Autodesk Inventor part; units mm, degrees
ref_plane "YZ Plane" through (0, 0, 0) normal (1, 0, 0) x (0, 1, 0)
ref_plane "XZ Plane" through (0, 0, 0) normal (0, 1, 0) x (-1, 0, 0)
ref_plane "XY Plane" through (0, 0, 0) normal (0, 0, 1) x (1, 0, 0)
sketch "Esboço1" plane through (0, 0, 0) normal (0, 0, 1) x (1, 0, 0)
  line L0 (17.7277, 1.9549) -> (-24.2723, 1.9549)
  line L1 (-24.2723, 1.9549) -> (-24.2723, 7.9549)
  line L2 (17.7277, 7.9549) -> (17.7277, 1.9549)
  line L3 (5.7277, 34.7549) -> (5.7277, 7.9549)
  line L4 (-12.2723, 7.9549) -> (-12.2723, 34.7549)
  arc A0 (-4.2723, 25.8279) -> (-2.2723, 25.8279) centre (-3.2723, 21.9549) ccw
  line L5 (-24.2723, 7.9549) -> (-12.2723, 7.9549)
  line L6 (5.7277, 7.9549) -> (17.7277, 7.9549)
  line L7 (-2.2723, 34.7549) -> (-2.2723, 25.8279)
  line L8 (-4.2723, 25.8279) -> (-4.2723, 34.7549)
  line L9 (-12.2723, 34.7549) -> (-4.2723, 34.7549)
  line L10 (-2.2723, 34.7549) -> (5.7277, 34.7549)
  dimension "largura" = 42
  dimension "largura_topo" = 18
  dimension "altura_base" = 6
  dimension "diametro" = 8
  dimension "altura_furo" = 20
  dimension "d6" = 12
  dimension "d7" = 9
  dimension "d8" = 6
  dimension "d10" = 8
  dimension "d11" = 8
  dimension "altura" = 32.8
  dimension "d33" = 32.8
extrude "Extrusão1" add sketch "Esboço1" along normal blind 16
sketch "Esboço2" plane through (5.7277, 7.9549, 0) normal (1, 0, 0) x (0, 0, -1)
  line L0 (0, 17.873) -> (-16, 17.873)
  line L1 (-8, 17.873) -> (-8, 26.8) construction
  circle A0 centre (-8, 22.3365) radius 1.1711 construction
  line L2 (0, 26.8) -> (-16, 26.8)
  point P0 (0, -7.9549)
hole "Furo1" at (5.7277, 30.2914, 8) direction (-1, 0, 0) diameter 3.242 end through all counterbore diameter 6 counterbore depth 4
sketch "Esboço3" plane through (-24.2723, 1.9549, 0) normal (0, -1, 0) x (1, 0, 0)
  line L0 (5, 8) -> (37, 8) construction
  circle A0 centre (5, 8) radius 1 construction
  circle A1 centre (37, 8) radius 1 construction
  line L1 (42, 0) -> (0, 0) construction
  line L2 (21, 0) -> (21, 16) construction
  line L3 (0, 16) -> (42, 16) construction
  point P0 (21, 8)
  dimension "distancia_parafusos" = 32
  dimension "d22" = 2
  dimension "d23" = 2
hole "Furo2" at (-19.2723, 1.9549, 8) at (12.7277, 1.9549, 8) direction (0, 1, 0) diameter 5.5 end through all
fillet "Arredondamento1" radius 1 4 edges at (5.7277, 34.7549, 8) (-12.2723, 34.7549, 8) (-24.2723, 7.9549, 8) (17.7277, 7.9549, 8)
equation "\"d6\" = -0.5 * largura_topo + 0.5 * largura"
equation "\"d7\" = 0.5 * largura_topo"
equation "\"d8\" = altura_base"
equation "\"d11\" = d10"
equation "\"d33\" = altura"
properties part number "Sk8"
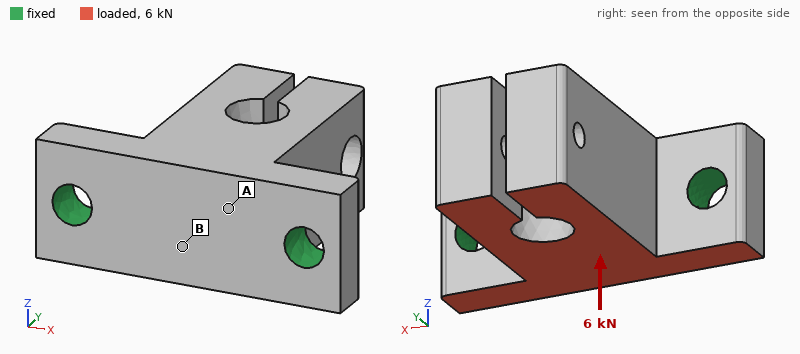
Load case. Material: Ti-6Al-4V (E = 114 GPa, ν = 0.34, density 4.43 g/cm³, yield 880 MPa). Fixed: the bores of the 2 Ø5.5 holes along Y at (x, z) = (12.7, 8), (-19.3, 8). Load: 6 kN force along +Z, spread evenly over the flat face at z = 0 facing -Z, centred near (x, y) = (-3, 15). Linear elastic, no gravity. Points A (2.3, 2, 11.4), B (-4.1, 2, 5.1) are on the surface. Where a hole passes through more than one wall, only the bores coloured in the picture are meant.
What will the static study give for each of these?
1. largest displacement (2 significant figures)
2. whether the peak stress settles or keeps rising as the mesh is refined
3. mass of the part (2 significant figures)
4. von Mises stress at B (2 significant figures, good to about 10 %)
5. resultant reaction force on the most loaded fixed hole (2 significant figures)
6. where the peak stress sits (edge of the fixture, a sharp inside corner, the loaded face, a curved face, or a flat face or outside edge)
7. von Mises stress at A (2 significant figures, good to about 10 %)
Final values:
0.18 mm
keeps rising
45 g
43 MPa
3.0 kN
edge of the fixture
82 MPa
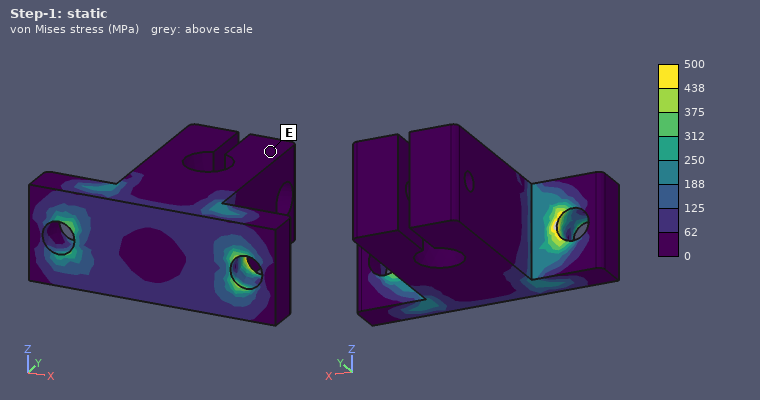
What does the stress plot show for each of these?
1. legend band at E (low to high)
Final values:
0 to 62 MPa
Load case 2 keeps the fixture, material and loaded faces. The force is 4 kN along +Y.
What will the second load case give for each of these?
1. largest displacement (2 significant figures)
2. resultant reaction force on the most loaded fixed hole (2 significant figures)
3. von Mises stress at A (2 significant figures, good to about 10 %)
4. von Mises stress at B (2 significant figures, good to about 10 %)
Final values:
79 µm
2.1 kN
37 MPa
35 MPa
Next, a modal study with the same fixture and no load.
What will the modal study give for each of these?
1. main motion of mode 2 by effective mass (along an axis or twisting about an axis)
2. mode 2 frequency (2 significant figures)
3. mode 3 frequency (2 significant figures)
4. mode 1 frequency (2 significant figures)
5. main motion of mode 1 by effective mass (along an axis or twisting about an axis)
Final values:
along X
8400 Hz
10 kHz
5300 Hz
along Z
